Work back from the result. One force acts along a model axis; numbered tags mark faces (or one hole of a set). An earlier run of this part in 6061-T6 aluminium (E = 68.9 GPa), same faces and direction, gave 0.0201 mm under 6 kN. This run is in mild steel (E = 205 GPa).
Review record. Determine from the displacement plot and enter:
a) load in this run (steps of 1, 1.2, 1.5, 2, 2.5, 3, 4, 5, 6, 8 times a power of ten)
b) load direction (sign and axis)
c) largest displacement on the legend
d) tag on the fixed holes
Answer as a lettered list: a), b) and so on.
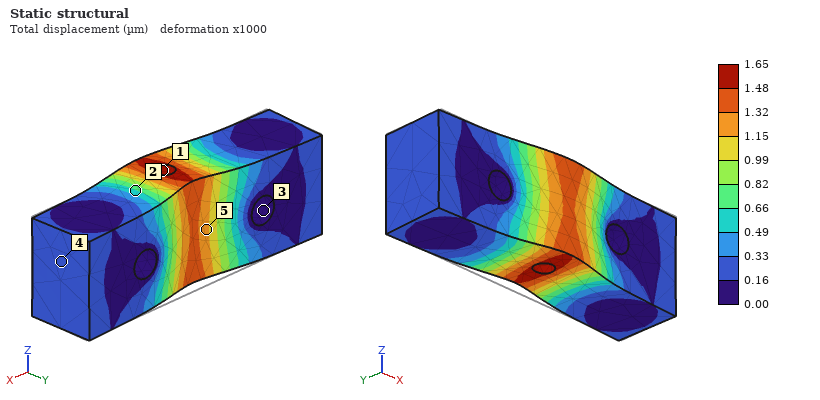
a) 1.5 kN
b) -Y
c) 1.65 µm
d) 3
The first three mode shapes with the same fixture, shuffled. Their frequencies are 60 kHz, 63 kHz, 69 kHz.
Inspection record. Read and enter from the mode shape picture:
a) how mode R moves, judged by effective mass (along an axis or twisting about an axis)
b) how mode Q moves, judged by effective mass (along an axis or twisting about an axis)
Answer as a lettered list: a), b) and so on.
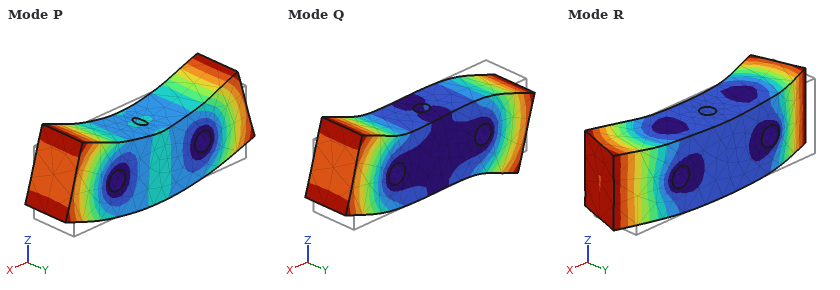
a) along Y
b) twisting about Y
